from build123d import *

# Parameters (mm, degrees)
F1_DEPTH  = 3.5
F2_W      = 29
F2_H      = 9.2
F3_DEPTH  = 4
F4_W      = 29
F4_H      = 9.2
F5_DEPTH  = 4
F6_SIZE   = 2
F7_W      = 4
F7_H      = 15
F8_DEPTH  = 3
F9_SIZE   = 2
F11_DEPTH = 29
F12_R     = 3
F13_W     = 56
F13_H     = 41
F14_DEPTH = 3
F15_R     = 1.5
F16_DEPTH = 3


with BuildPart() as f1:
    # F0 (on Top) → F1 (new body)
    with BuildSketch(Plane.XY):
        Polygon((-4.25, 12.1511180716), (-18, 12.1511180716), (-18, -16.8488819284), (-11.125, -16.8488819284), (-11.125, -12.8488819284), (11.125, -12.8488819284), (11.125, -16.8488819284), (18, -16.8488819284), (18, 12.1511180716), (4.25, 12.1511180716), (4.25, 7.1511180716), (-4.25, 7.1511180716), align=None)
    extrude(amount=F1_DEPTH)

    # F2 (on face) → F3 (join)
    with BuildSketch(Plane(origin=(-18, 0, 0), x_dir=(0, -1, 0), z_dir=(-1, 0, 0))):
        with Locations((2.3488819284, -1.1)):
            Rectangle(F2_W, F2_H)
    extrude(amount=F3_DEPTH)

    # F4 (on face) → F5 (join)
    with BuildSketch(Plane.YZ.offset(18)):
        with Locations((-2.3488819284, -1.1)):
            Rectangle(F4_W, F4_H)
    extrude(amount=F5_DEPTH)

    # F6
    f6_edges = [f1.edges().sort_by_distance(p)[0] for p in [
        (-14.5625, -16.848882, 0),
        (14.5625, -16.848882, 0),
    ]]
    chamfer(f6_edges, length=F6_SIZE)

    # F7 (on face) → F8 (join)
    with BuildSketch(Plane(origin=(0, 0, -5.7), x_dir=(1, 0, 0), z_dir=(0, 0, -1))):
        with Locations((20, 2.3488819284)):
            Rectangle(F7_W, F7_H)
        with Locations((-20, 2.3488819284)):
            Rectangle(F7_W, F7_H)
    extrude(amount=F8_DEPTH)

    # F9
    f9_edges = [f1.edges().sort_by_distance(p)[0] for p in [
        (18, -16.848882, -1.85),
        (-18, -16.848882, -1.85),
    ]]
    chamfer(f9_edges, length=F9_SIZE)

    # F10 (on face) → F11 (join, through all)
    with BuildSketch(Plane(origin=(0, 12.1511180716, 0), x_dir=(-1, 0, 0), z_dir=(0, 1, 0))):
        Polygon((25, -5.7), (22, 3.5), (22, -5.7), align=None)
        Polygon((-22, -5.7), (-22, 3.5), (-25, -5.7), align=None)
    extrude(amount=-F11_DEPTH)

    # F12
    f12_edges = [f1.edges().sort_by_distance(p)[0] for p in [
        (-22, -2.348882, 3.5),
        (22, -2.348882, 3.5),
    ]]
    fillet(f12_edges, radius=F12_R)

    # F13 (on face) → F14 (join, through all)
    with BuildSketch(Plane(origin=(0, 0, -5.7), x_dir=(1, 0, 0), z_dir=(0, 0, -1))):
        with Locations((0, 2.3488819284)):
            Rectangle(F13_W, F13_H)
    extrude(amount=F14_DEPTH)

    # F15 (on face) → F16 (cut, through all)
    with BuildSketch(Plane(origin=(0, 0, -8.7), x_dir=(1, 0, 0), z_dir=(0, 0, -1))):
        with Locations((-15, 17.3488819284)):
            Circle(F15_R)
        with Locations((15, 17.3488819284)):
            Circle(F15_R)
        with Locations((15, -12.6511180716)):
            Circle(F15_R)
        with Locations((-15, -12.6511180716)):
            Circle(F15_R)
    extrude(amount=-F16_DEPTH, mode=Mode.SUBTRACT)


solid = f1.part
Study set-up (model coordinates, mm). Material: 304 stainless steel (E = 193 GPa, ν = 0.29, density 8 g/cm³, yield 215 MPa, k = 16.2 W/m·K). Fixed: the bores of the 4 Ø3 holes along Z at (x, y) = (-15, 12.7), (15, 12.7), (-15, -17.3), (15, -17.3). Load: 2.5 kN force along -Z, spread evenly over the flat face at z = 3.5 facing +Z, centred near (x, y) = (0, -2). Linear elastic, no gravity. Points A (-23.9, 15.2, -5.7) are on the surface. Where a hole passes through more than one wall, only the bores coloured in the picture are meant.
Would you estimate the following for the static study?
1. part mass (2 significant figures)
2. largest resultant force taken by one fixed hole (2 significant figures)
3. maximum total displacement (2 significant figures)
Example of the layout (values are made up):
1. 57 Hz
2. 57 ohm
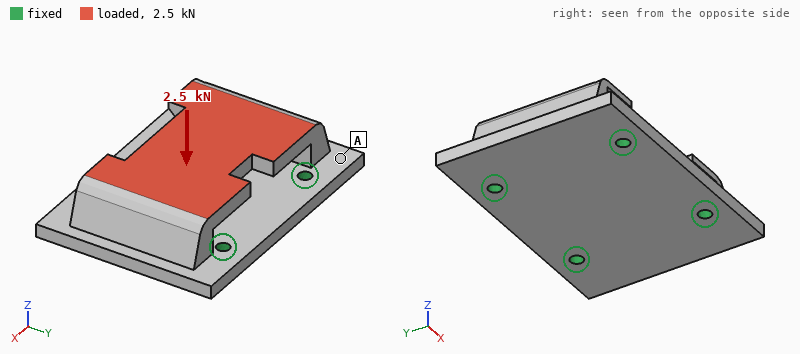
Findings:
1. 100 g
2. 670 N
3. 32 µm
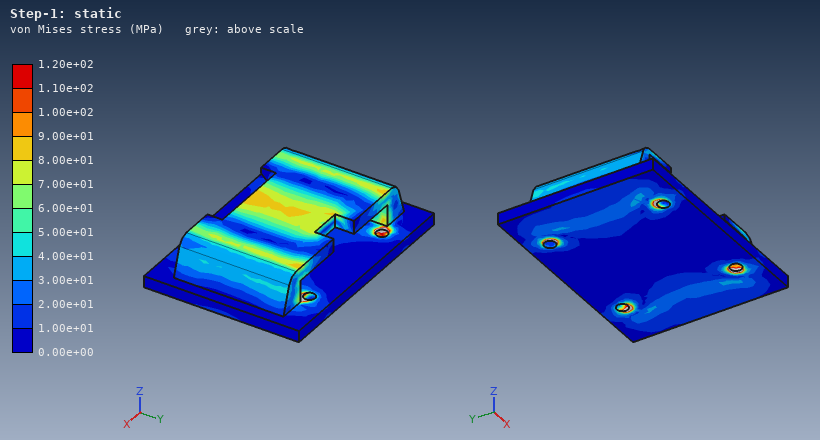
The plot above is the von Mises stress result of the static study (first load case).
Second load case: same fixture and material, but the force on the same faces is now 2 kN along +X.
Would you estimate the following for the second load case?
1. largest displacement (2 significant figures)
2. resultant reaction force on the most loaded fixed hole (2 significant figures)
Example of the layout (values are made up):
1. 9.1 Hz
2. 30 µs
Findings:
1. 21 µm
2. 560 N
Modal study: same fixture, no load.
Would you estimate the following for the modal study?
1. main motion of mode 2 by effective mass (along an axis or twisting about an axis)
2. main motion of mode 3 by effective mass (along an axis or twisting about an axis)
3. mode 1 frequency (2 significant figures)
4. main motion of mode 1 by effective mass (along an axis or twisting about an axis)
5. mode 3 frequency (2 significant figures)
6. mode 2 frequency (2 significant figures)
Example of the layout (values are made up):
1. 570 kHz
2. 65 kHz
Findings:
1. along Z
2. along Z
3. 7600 Hz
4. along X
5. 13 kHz
6. 9600 Hz
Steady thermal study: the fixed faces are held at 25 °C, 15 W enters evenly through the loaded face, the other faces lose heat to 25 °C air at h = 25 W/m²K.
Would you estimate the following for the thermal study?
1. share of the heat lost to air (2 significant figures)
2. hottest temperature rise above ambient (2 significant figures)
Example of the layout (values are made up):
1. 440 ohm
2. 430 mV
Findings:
1. 32 %
2. 82 K
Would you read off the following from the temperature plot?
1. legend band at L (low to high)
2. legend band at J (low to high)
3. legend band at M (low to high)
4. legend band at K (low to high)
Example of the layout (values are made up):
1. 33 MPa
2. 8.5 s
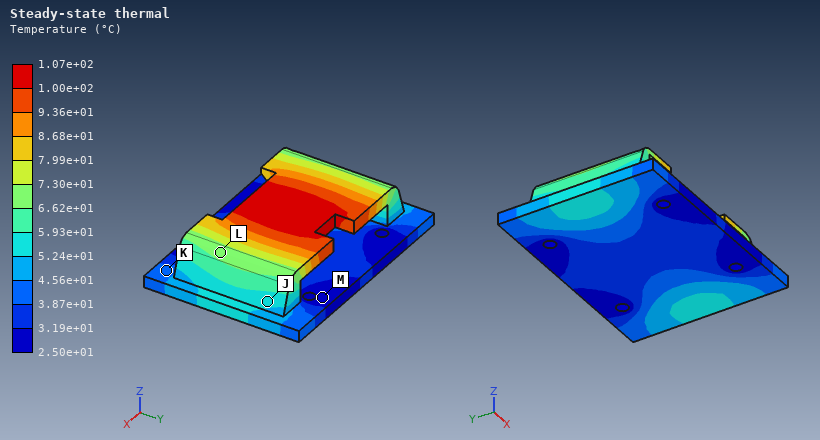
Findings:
1. 6.62e+01 to 7.30e+01 °C
2. 5.24e+01 to 5.93e+01 °C
3. 2.50e+01 to 3.19e+01 °C
4. 3.87e+01 to 4.56e+01 °C
